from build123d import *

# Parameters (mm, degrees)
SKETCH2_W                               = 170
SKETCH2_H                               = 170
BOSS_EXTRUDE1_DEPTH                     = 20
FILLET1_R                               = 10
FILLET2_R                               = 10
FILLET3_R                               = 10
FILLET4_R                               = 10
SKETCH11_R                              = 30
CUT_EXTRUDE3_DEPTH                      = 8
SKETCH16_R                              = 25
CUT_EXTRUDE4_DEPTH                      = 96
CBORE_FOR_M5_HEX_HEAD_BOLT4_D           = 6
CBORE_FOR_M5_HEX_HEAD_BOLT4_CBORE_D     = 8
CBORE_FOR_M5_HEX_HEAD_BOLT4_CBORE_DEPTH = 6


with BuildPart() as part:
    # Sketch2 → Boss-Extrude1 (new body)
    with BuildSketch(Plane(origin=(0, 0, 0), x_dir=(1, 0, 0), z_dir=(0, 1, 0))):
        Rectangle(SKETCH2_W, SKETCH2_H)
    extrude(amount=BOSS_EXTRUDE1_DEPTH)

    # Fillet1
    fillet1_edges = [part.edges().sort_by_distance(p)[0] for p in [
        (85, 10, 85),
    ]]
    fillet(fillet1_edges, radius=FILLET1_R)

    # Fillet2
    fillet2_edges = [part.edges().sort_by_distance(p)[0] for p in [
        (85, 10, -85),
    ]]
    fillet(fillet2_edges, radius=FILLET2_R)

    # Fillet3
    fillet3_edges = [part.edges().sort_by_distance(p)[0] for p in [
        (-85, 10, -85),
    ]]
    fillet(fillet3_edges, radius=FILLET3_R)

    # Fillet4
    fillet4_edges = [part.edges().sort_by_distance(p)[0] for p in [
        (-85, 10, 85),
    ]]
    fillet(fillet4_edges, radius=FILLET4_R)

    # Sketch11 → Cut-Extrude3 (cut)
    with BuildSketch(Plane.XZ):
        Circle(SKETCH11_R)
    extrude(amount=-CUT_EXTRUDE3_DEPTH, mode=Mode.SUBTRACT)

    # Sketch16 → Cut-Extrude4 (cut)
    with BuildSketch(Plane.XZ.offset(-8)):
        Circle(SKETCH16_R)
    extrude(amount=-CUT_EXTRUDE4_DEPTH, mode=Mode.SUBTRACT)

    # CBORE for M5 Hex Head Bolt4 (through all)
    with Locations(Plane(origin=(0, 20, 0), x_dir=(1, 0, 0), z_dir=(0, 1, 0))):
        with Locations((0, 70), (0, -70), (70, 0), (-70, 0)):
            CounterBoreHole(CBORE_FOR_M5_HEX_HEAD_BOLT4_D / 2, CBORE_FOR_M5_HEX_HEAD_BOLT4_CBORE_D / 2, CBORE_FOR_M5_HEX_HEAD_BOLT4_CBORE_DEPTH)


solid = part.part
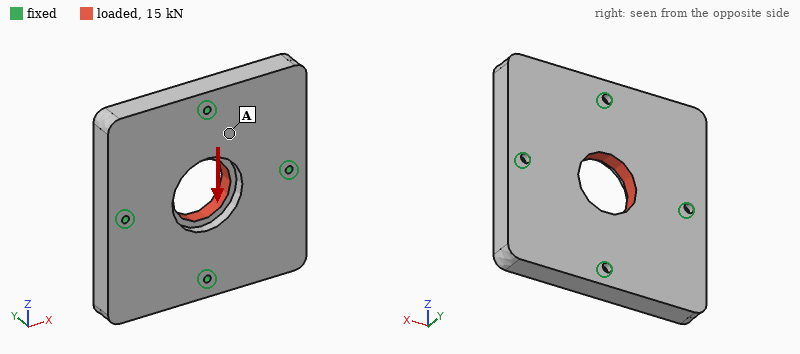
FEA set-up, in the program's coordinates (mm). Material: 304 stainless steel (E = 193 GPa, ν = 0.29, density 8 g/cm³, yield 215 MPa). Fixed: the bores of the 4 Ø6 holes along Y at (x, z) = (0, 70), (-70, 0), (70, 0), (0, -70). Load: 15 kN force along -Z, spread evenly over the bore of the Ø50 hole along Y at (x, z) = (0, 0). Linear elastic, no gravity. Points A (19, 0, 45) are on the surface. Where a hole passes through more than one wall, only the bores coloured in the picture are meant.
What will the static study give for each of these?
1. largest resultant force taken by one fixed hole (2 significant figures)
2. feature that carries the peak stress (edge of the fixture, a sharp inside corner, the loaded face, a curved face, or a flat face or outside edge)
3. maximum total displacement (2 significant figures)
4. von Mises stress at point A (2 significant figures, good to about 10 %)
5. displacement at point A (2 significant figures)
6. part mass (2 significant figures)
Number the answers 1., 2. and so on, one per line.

1. 4.4 kN
2. edge of the fixture
3. 2.5 µm
4. 3.1 MPa
5. 1.1 µm
6. 4.2 kg
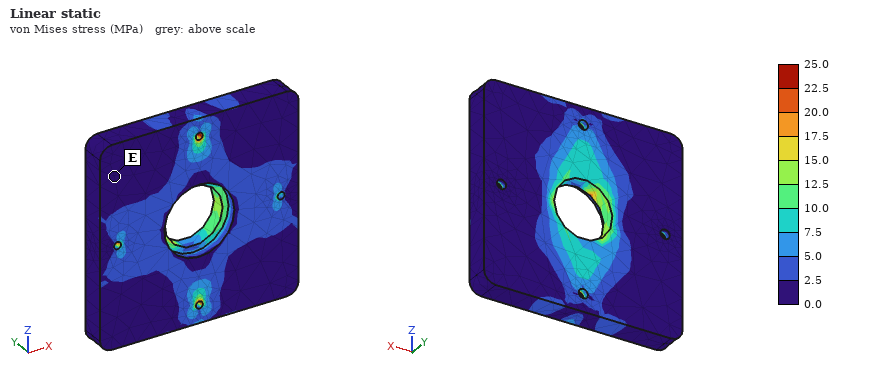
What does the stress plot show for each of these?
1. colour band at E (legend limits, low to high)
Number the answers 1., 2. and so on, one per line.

1. 0.0 to 2.5 MPa
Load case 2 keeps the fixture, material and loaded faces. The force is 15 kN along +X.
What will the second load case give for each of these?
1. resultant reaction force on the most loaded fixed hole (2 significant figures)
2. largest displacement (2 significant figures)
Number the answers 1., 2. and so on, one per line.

1. 4.4 kN
2. 2.5 µm
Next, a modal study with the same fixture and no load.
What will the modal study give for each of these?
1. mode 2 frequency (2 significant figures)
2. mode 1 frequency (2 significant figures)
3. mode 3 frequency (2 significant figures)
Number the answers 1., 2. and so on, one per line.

1. 3400 Hz
2. 2800 Hz
3. 3400 Hz
